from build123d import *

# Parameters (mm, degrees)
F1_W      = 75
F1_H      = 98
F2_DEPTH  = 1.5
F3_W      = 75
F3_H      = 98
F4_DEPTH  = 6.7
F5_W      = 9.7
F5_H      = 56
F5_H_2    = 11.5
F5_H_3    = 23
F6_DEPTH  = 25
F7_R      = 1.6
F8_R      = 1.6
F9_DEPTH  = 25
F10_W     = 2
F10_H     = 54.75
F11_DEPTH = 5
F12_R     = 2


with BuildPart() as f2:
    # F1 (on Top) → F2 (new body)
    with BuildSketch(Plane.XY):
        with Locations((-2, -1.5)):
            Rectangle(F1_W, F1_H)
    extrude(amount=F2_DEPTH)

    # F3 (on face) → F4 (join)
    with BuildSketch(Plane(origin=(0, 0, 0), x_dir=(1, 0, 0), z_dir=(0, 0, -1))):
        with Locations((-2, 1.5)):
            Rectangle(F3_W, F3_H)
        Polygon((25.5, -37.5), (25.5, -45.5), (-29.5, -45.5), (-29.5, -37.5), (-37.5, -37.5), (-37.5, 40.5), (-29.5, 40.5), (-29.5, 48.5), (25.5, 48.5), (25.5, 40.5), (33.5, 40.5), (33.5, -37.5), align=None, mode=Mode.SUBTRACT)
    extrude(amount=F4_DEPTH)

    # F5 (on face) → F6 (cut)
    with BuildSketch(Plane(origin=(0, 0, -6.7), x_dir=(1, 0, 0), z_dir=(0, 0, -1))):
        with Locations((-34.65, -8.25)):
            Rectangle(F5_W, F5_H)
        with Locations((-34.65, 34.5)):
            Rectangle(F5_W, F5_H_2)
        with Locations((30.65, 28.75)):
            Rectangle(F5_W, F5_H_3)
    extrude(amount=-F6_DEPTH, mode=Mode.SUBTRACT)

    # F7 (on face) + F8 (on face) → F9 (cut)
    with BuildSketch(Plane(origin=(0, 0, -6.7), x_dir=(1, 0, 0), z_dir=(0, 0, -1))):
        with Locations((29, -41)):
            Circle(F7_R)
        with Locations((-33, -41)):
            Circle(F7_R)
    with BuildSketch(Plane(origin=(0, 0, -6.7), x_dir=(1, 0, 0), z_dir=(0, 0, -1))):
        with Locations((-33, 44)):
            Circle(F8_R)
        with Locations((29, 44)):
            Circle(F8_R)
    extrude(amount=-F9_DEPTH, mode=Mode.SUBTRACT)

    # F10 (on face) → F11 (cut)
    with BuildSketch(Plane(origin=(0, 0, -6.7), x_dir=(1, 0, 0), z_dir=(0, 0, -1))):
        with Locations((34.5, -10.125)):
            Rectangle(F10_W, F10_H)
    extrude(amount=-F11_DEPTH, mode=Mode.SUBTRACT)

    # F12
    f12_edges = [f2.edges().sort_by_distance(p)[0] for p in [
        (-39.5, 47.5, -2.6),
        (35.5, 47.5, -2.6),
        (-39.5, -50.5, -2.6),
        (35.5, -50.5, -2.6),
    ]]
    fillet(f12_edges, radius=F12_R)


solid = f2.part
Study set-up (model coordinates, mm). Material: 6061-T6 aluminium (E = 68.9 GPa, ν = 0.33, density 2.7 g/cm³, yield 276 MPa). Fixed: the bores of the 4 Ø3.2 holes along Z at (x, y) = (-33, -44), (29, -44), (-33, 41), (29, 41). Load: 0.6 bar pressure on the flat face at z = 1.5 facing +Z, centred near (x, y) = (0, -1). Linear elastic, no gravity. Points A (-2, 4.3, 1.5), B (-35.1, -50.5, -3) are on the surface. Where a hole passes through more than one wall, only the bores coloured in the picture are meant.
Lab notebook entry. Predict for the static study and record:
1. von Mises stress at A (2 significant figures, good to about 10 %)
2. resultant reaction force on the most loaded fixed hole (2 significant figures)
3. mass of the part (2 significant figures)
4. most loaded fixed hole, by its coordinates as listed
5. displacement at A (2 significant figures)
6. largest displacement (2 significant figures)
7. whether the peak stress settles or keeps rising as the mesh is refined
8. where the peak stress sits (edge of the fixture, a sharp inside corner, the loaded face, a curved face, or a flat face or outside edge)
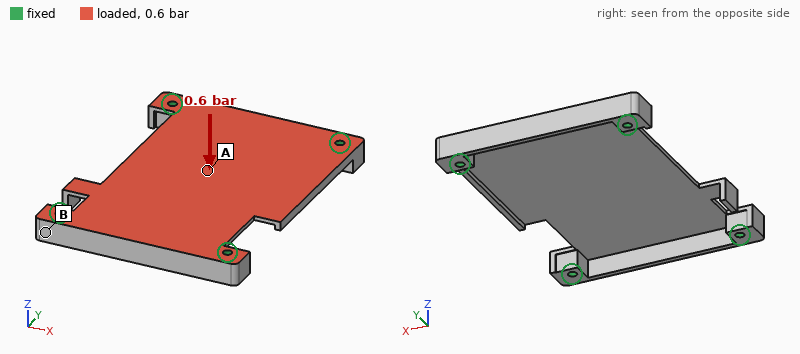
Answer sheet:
43 MPa
150 N
38 g
(29, 41)
0.52 mm
0.60 mm
keeps rising
a sharp inside corner
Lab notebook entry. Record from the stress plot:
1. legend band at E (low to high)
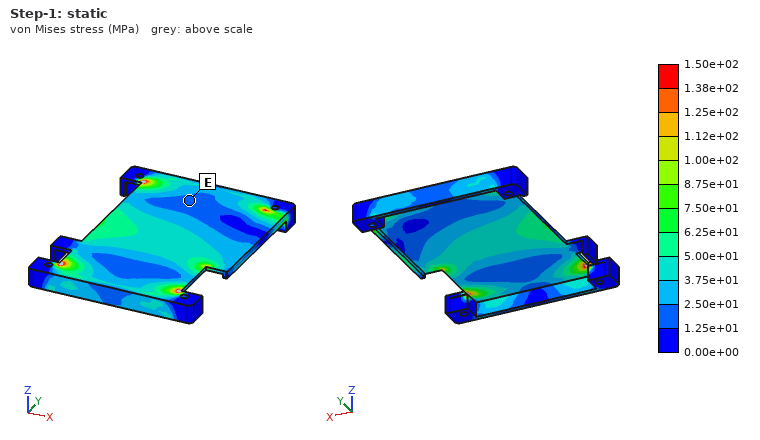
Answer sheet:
1.25e+01 to 2.50e+01 MPa
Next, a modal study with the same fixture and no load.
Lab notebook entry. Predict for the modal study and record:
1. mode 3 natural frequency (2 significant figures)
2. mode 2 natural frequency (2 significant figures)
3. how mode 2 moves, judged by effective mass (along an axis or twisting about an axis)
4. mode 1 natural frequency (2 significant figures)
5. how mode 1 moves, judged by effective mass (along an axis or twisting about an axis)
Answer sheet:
2100 Hz
1400 Hz
twisting about Y
950 Hz
along Z
